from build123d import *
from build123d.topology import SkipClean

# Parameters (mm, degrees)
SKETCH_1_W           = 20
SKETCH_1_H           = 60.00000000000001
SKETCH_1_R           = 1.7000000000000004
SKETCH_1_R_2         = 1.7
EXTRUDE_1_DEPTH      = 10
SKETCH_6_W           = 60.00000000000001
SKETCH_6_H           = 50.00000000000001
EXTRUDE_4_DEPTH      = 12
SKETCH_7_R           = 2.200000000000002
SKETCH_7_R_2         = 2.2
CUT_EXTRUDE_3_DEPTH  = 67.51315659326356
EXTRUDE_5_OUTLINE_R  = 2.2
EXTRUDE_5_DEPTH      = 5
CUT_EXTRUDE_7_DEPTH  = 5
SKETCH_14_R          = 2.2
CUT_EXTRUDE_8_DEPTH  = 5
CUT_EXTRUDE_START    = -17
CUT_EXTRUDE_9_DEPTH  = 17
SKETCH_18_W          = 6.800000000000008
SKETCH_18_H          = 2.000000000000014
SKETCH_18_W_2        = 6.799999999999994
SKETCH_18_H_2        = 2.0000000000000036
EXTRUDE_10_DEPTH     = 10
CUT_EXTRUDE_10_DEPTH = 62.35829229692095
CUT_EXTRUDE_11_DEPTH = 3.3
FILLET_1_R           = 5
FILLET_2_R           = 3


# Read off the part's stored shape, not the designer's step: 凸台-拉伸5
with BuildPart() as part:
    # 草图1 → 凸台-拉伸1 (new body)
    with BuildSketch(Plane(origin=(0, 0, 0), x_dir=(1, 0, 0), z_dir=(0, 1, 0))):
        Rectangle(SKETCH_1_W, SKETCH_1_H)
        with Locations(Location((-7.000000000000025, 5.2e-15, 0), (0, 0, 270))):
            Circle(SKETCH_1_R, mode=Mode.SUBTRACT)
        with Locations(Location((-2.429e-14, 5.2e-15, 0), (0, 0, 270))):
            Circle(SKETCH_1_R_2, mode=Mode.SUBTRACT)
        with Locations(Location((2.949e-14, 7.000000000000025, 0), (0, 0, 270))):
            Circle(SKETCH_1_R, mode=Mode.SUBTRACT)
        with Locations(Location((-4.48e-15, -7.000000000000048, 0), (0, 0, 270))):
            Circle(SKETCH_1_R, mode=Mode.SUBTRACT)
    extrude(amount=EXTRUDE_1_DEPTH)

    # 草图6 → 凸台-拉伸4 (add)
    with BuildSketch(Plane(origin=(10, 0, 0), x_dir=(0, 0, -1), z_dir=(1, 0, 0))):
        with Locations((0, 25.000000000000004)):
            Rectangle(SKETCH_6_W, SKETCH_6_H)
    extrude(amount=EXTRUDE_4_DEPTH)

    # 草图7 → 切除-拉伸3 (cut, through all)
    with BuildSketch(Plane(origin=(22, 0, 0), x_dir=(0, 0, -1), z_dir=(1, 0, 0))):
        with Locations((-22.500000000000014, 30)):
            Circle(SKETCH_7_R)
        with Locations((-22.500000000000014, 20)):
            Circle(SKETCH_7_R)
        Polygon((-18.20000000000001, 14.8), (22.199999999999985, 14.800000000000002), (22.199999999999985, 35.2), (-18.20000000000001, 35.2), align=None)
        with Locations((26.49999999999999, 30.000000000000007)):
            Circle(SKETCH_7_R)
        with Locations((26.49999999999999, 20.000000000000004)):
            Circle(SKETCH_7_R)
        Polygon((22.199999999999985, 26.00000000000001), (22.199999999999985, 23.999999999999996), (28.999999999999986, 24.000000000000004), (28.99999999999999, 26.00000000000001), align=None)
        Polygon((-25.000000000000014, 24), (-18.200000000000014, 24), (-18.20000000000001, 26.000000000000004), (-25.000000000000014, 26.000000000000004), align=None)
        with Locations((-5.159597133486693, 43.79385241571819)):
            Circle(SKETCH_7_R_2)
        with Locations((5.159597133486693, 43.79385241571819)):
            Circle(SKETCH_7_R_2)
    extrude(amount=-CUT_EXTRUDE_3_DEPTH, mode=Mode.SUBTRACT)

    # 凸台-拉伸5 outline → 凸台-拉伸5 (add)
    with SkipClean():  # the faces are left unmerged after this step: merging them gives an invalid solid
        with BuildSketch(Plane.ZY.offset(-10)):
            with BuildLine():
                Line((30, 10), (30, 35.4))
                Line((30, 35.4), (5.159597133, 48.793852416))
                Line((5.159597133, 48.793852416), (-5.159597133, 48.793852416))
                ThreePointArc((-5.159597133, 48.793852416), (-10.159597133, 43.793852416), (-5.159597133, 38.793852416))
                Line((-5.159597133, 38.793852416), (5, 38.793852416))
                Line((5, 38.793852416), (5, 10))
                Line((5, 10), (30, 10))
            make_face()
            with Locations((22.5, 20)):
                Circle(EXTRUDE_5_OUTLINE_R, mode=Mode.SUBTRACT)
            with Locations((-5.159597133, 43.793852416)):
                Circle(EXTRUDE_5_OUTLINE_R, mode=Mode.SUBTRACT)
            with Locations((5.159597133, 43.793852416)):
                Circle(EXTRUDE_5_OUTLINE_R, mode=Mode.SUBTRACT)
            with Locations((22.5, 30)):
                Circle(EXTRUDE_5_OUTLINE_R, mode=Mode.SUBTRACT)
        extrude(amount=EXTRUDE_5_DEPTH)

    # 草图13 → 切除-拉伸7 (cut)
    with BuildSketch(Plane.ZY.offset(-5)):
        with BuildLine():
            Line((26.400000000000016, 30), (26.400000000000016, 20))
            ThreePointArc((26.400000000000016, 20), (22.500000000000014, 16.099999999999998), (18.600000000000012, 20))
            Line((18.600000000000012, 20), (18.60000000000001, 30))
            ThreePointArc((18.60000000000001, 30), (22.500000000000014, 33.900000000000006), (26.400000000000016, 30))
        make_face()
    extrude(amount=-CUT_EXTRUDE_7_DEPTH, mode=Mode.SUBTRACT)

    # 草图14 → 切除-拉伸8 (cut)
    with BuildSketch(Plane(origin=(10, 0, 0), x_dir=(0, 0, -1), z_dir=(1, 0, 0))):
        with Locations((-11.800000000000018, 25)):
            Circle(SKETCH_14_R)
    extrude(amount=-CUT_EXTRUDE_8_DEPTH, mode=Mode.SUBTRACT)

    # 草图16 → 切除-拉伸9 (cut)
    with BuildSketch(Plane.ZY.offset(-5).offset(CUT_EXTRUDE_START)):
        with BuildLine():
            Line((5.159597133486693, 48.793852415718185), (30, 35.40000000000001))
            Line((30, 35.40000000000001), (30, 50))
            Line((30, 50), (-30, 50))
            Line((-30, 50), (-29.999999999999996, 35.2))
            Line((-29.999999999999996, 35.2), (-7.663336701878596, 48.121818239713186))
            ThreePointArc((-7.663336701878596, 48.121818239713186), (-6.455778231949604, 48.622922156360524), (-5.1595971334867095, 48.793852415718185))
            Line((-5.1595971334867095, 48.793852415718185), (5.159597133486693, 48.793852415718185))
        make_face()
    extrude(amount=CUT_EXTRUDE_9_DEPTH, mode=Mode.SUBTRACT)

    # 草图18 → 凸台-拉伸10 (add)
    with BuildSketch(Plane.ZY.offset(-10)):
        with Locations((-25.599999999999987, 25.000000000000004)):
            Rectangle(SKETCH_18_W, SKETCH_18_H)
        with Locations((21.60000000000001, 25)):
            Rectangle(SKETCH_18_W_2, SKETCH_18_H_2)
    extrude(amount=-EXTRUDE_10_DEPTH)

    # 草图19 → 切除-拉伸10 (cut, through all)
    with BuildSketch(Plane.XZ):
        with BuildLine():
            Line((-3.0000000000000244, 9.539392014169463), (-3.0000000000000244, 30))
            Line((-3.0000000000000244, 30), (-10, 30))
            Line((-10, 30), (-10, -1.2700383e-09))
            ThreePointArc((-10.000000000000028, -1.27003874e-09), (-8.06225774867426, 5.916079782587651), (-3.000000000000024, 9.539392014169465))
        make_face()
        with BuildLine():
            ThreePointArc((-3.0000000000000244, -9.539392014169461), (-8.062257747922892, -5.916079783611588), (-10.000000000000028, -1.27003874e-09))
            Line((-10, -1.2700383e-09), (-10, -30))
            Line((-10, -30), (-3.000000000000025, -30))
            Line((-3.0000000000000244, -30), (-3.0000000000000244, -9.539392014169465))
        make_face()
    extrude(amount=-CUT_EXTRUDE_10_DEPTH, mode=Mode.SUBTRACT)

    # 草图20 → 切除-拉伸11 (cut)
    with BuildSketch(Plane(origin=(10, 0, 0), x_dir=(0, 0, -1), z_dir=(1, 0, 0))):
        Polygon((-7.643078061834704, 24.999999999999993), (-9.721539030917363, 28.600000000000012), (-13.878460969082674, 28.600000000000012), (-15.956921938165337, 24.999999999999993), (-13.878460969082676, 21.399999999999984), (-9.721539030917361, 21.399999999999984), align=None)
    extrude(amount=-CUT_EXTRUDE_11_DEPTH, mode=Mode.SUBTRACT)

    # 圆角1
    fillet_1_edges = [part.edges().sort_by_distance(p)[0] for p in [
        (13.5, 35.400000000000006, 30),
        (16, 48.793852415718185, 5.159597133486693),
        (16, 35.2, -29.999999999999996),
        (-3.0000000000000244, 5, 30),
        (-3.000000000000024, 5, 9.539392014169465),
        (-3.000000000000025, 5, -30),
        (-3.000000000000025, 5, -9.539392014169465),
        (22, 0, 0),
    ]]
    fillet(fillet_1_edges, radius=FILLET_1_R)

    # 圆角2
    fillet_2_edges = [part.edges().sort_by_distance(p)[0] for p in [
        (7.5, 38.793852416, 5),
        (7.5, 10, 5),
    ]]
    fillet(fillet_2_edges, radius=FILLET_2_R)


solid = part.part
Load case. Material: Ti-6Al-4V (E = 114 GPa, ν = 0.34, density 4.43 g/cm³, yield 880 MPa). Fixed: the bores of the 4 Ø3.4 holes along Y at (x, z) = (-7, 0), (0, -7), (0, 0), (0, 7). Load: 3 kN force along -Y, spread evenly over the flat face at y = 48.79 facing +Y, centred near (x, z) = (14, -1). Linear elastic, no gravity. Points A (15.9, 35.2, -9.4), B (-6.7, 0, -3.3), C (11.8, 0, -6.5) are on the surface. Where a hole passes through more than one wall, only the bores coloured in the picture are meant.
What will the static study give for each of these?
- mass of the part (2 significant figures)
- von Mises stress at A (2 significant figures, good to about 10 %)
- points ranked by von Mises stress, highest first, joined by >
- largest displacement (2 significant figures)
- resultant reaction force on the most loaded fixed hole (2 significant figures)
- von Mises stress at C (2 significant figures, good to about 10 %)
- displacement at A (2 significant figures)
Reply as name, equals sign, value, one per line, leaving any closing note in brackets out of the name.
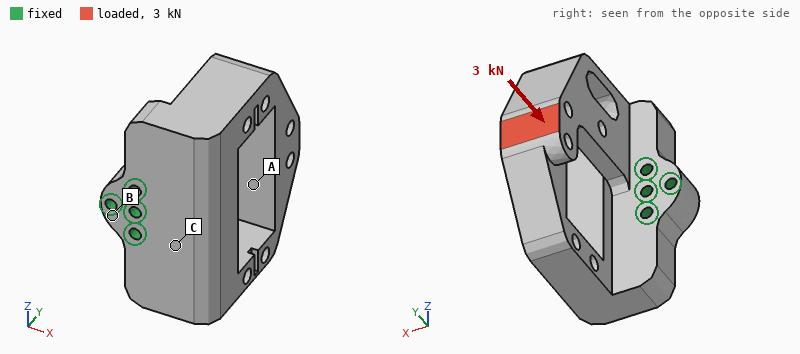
mass of the part = 140 g
von Mises stress at A = 45 MPa
points ranked by von Mises stress, highest first, joined by > = A > C > B
largest displacement = 78 µm
resultant reaction force on the most loaded fixed hole = 1.3 kN
von Mises stress at C = 25 MPa
displacement at A = 54 µm
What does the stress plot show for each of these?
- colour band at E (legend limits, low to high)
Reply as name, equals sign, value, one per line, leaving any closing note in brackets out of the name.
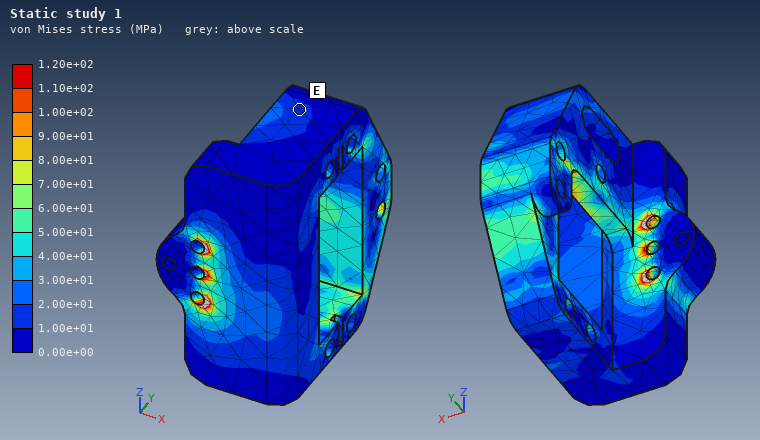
colour band at E = 1.00e+01 to 2.00e+01 MPa
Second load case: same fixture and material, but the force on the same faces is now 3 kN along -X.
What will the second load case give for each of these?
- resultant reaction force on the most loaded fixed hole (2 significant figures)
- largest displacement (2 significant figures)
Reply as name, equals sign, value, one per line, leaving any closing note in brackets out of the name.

resultant reaction force on the most loaded fixed hole = 1.6 kN
largest displacement = 0.44 mm
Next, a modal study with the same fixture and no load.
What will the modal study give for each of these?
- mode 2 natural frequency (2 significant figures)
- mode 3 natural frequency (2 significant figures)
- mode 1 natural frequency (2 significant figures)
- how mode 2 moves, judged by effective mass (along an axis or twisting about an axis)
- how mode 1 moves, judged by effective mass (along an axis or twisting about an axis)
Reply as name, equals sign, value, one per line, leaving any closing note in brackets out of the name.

mode 2 natural frequency = 3600 Hz
mode 3 natural frequency = 5900 Hz
mode 1 natural frequency = 2700 Hz
how mode 2 moves, judged by effective mass = along Z
how mode 1 moves, judged by effective mass = along X
